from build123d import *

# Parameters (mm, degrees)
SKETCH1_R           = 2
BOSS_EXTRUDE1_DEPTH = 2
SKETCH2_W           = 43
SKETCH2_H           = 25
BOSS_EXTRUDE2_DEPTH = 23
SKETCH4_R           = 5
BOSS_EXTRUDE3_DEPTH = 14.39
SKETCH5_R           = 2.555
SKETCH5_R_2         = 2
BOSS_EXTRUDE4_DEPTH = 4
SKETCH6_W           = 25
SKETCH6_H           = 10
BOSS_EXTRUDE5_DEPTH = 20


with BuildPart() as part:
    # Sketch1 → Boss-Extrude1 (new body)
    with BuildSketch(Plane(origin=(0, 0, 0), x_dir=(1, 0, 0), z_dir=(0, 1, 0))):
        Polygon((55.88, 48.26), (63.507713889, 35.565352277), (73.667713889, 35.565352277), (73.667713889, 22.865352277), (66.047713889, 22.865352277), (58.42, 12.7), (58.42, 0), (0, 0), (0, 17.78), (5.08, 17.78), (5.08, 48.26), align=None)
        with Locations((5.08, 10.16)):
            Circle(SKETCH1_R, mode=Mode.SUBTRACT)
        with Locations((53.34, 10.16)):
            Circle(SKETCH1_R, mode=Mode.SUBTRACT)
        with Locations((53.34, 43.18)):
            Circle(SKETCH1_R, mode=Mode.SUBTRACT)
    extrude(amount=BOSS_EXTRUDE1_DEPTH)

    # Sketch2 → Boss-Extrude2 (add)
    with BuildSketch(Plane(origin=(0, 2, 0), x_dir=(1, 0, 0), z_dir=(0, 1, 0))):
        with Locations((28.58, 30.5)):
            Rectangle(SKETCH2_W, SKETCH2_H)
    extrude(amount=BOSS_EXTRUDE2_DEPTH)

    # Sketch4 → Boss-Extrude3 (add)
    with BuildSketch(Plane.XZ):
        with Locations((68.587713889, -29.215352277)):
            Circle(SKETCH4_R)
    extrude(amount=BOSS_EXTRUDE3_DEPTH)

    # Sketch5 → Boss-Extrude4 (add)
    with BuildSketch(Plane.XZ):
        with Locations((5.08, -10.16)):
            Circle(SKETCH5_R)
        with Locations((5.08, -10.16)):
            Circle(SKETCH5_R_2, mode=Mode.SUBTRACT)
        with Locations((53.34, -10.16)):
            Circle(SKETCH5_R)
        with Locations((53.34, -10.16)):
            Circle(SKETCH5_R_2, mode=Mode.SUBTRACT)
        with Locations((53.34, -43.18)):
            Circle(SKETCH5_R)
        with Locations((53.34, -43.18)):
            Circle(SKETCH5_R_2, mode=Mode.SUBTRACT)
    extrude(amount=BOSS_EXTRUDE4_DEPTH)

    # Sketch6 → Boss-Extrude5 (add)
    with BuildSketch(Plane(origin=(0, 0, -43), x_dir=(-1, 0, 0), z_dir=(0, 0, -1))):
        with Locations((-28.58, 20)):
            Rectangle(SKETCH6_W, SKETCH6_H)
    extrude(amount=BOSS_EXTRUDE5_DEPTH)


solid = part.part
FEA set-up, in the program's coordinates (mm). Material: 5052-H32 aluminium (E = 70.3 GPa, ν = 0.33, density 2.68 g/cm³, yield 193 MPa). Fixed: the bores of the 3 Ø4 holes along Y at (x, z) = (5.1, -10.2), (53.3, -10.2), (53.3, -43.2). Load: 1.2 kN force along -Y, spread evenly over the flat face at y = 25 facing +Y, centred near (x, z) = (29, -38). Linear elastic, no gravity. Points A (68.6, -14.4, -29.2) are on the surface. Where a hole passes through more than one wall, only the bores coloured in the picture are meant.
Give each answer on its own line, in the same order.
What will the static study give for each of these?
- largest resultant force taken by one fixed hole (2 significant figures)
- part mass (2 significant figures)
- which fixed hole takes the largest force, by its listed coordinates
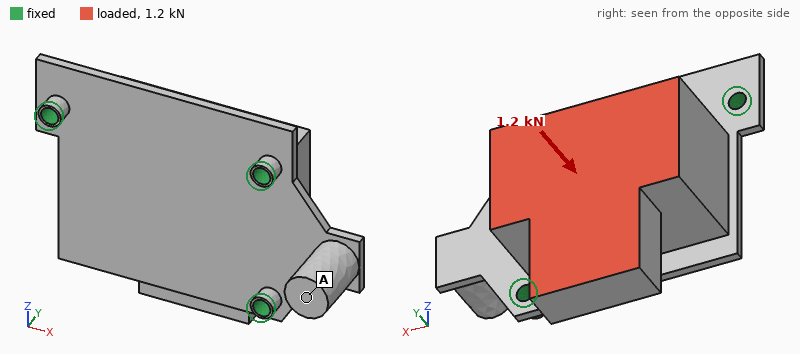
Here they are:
1.1 kN
98 g
(53.3, -43.2)
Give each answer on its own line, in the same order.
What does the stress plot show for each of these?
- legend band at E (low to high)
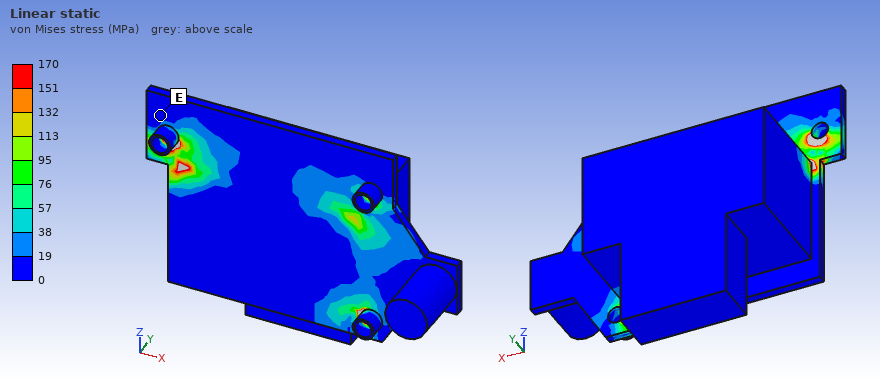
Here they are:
0 to 19 MPa
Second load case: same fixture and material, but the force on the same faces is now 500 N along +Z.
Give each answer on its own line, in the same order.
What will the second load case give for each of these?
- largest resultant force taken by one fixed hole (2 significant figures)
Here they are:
490 N
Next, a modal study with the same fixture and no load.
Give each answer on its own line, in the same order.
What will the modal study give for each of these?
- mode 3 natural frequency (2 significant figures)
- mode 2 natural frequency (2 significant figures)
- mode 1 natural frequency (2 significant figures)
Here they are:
3200 Hz
1800 Hz
1600 Hz
